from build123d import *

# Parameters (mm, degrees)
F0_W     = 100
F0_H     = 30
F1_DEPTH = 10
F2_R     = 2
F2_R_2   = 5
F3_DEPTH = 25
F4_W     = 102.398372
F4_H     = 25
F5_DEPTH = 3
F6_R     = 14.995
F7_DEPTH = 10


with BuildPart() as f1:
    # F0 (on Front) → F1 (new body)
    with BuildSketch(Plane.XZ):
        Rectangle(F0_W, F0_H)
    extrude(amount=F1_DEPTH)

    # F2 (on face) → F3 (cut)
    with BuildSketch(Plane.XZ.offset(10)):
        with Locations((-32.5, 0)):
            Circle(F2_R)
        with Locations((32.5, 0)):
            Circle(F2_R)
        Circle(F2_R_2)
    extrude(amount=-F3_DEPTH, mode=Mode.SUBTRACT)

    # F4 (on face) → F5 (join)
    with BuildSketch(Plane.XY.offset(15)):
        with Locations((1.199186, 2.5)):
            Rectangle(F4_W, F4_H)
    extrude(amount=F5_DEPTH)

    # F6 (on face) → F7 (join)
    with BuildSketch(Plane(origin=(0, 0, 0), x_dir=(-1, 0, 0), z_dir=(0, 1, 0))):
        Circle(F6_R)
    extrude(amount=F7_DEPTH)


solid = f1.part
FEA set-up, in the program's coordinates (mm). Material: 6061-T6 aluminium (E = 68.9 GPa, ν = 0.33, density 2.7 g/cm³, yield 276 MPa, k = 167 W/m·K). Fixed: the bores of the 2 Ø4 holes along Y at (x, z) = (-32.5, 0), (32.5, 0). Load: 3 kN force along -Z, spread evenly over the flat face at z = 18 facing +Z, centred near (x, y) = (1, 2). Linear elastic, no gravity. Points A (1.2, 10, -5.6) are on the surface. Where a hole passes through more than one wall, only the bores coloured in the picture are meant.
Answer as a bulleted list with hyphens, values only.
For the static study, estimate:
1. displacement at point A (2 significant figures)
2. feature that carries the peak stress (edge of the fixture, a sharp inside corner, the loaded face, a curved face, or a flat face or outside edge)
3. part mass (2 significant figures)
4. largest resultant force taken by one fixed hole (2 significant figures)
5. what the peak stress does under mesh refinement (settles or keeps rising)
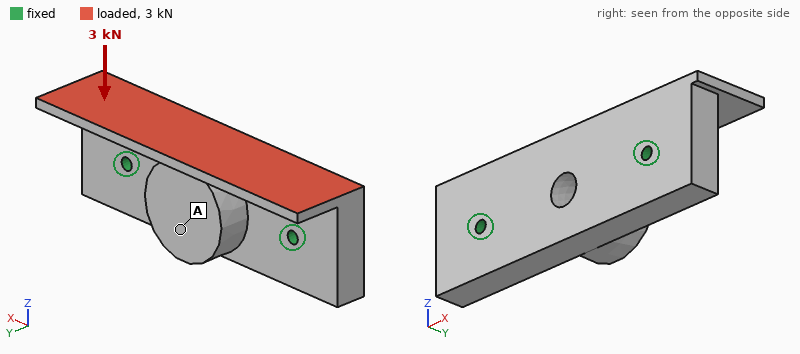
- 15 µm
- edge of the fixture
- 120 g
- 1.6 kN
- keeps rising
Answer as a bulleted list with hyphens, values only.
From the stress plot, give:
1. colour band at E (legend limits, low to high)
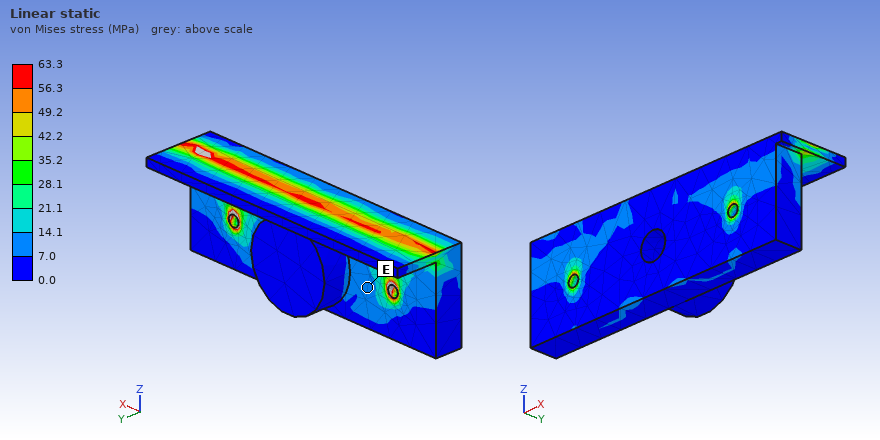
- 7.0 to 14.1 MPa
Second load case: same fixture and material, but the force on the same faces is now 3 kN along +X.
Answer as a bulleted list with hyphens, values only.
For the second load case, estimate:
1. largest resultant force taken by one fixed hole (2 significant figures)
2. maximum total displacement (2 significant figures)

- 1.7 kN
- 15 µm
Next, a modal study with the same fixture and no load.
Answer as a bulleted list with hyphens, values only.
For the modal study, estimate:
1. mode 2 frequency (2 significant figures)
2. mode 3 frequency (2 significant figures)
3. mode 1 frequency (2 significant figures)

- 8600 Hz
- 8800 Hz
- 6400 Hz
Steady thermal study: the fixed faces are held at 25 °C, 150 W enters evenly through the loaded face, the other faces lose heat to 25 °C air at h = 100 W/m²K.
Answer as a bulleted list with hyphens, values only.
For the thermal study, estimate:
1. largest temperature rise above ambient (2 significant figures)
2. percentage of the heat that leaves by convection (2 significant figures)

- 39 K
- 13 %
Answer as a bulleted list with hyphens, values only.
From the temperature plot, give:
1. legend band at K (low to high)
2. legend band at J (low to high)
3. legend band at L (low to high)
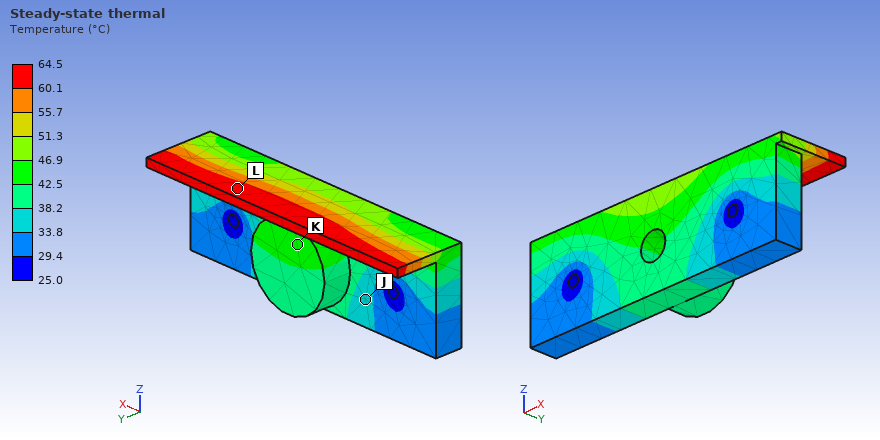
- 42.5 to 46.9 °C
- 33.8 to 38.2 °C
- 60.1 to 64.5 °C
